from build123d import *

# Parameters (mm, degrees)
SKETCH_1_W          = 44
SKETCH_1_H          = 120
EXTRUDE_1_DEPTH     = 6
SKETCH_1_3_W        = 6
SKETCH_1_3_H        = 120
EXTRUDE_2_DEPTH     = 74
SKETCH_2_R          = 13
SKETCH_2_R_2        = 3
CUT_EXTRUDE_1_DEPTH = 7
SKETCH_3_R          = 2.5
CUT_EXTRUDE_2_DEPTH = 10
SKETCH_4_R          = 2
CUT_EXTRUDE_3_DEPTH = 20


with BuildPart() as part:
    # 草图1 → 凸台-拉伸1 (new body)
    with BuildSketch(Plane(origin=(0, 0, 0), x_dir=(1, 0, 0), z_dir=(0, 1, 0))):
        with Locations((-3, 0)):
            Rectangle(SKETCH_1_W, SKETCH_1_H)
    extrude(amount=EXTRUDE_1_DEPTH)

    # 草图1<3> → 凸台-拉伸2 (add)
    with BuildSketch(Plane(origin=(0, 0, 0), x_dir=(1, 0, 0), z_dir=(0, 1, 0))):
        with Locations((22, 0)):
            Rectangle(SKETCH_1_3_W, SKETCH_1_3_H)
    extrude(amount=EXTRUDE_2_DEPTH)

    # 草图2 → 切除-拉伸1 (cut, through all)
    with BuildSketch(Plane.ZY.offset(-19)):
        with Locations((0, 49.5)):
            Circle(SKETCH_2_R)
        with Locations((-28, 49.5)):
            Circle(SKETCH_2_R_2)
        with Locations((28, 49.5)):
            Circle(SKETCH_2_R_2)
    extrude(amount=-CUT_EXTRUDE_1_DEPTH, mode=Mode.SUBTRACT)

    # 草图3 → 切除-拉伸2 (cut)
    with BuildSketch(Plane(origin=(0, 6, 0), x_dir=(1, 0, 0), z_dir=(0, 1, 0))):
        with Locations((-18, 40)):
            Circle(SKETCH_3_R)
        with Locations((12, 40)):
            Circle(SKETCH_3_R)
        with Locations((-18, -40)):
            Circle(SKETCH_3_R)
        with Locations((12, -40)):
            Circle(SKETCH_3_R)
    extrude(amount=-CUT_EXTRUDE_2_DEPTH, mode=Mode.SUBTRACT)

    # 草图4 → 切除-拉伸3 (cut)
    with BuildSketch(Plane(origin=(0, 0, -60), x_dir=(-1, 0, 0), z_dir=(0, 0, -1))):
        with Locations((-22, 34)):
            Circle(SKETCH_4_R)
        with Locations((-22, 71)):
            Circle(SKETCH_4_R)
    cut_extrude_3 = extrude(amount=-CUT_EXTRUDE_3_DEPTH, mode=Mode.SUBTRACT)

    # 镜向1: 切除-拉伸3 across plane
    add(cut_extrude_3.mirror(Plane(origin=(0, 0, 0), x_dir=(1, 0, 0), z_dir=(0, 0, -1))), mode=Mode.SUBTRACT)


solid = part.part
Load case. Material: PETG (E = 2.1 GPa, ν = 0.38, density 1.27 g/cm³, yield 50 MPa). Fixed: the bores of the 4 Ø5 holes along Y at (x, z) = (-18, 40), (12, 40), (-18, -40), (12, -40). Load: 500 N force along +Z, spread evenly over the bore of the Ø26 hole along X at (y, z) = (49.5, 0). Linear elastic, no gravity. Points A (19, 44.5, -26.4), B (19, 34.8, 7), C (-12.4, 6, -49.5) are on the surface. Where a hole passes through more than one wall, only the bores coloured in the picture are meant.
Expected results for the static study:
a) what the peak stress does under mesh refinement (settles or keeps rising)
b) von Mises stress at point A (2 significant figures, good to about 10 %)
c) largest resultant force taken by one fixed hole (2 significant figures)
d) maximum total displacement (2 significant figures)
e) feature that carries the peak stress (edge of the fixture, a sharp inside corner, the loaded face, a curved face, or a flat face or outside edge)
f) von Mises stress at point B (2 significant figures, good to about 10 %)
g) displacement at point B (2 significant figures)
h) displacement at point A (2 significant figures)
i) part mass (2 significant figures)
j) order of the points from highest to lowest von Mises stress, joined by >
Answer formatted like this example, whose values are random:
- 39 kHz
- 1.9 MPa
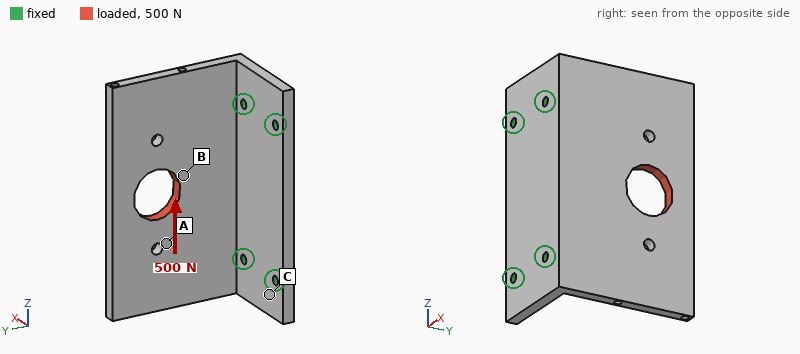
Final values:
- keeps rising
- 2.4 MPa
- 370 N
- 0.50 mm
- edge of the fixture
- 3.4 MPa
- 0.14 mm
- 0.23 mm
- 100 g
- B > A > C
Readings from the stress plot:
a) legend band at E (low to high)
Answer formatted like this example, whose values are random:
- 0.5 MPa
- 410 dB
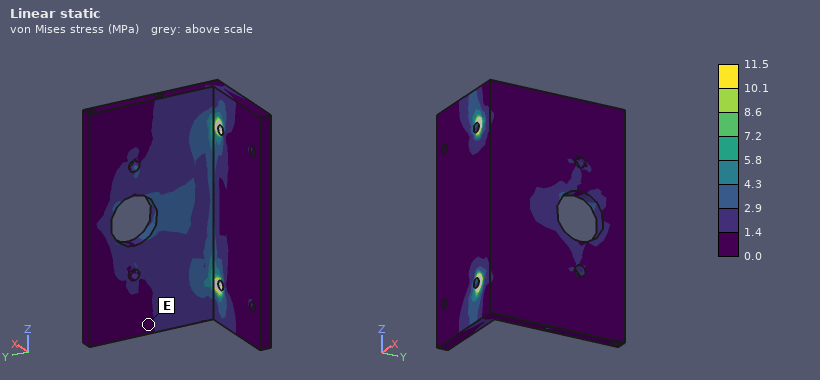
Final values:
- 0.0 to 1.4 MPa
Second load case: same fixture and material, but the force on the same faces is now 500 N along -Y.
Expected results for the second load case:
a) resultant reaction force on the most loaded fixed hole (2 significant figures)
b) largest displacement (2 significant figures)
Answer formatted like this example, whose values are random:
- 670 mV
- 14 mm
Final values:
- 290 N
- 0.64 mm
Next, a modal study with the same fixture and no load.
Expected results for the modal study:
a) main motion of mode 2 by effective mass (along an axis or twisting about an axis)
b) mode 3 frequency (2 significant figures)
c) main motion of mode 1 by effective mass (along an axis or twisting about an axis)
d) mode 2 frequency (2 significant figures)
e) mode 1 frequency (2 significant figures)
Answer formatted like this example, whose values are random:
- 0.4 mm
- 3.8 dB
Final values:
- twisting about Y
- 820 Hz
- along X
- 360 Hz
- 210 Hz
